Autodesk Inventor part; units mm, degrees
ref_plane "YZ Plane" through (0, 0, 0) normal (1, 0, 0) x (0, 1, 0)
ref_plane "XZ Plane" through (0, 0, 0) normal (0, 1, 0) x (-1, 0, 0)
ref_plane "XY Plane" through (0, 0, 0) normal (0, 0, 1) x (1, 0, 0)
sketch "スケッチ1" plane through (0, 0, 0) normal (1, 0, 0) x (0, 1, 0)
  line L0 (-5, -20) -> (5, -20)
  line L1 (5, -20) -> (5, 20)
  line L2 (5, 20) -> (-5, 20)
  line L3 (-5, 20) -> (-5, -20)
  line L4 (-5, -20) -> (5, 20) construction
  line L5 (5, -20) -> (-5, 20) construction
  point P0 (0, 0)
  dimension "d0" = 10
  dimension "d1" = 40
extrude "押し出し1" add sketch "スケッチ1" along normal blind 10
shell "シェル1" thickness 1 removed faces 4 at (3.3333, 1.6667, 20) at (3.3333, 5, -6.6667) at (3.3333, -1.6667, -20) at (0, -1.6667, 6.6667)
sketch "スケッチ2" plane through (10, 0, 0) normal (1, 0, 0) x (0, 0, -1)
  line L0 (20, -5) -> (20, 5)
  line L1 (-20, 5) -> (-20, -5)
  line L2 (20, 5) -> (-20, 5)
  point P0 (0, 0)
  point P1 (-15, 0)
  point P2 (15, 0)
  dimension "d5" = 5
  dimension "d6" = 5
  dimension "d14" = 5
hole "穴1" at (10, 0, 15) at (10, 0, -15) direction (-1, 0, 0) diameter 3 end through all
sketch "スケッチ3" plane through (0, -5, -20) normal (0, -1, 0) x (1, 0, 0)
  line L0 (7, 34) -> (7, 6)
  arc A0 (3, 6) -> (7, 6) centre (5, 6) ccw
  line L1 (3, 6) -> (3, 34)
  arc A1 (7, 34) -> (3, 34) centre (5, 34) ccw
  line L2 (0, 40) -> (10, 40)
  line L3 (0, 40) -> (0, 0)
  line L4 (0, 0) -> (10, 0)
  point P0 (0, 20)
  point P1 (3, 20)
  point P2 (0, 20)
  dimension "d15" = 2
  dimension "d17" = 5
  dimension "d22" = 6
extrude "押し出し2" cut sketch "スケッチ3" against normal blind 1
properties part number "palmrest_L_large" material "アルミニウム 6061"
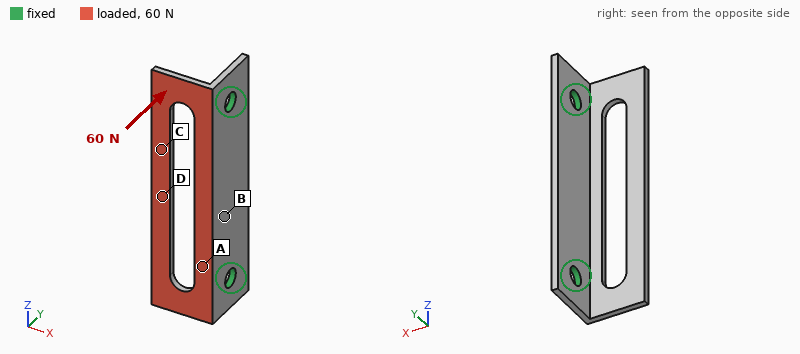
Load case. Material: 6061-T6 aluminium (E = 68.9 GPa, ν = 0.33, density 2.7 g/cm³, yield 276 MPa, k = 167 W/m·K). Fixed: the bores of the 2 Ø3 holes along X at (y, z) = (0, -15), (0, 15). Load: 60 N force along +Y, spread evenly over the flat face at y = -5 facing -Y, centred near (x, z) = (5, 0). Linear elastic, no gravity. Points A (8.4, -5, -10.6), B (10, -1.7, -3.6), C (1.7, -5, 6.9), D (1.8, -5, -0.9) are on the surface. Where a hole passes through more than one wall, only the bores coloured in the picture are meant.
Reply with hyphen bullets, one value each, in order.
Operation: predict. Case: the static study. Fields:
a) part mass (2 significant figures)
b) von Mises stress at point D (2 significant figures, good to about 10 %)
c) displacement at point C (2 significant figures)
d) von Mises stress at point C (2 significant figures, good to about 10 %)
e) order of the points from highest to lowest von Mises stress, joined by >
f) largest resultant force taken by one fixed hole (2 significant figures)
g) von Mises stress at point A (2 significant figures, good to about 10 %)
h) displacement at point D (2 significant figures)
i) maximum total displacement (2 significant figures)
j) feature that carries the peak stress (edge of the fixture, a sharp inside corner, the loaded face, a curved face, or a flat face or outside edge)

- 1.7 g
- 80 MPa
- 0.29 mm
- 49 MPa
- D > C > A > B
- 30 N
- 30 MPa
- 0.34 mm
- 0.38 mm
- a curved face
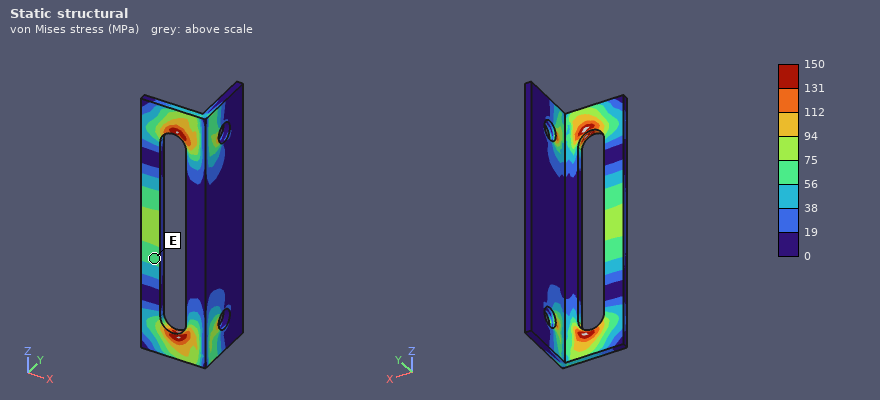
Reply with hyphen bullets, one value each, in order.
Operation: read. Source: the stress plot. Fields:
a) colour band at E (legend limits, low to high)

- 56 to 75 MPa
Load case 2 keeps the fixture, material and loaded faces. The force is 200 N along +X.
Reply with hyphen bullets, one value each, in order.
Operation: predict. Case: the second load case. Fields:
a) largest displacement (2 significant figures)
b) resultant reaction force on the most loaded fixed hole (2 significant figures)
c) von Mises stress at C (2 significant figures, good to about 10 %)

- 0.20 mm
- 100 N
- 30 MPa
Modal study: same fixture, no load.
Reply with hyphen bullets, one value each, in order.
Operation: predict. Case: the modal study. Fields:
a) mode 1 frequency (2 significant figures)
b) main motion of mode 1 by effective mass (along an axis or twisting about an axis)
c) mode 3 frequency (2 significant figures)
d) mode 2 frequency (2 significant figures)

- 2800 Hz
- along Y
- 7100 Hz
- 5700 Hz
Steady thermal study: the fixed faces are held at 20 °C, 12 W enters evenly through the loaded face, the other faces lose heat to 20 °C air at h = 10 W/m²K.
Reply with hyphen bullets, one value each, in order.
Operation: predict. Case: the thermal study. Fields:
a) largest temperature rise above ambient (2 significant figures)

- 76 K
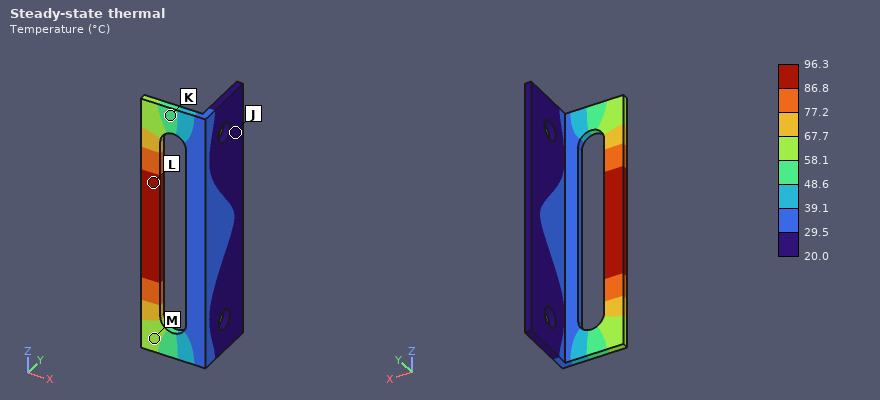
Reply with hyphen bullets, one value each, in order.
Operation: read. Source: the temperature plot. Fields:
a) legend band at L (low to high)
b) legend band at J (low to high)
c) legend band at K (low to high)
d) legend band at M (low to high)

- 86.8 to 96.3 °C
- 20.0 to 29.5 °C
- 48.6 to 58.1 °C
- 58.1 to 67.7 °C
